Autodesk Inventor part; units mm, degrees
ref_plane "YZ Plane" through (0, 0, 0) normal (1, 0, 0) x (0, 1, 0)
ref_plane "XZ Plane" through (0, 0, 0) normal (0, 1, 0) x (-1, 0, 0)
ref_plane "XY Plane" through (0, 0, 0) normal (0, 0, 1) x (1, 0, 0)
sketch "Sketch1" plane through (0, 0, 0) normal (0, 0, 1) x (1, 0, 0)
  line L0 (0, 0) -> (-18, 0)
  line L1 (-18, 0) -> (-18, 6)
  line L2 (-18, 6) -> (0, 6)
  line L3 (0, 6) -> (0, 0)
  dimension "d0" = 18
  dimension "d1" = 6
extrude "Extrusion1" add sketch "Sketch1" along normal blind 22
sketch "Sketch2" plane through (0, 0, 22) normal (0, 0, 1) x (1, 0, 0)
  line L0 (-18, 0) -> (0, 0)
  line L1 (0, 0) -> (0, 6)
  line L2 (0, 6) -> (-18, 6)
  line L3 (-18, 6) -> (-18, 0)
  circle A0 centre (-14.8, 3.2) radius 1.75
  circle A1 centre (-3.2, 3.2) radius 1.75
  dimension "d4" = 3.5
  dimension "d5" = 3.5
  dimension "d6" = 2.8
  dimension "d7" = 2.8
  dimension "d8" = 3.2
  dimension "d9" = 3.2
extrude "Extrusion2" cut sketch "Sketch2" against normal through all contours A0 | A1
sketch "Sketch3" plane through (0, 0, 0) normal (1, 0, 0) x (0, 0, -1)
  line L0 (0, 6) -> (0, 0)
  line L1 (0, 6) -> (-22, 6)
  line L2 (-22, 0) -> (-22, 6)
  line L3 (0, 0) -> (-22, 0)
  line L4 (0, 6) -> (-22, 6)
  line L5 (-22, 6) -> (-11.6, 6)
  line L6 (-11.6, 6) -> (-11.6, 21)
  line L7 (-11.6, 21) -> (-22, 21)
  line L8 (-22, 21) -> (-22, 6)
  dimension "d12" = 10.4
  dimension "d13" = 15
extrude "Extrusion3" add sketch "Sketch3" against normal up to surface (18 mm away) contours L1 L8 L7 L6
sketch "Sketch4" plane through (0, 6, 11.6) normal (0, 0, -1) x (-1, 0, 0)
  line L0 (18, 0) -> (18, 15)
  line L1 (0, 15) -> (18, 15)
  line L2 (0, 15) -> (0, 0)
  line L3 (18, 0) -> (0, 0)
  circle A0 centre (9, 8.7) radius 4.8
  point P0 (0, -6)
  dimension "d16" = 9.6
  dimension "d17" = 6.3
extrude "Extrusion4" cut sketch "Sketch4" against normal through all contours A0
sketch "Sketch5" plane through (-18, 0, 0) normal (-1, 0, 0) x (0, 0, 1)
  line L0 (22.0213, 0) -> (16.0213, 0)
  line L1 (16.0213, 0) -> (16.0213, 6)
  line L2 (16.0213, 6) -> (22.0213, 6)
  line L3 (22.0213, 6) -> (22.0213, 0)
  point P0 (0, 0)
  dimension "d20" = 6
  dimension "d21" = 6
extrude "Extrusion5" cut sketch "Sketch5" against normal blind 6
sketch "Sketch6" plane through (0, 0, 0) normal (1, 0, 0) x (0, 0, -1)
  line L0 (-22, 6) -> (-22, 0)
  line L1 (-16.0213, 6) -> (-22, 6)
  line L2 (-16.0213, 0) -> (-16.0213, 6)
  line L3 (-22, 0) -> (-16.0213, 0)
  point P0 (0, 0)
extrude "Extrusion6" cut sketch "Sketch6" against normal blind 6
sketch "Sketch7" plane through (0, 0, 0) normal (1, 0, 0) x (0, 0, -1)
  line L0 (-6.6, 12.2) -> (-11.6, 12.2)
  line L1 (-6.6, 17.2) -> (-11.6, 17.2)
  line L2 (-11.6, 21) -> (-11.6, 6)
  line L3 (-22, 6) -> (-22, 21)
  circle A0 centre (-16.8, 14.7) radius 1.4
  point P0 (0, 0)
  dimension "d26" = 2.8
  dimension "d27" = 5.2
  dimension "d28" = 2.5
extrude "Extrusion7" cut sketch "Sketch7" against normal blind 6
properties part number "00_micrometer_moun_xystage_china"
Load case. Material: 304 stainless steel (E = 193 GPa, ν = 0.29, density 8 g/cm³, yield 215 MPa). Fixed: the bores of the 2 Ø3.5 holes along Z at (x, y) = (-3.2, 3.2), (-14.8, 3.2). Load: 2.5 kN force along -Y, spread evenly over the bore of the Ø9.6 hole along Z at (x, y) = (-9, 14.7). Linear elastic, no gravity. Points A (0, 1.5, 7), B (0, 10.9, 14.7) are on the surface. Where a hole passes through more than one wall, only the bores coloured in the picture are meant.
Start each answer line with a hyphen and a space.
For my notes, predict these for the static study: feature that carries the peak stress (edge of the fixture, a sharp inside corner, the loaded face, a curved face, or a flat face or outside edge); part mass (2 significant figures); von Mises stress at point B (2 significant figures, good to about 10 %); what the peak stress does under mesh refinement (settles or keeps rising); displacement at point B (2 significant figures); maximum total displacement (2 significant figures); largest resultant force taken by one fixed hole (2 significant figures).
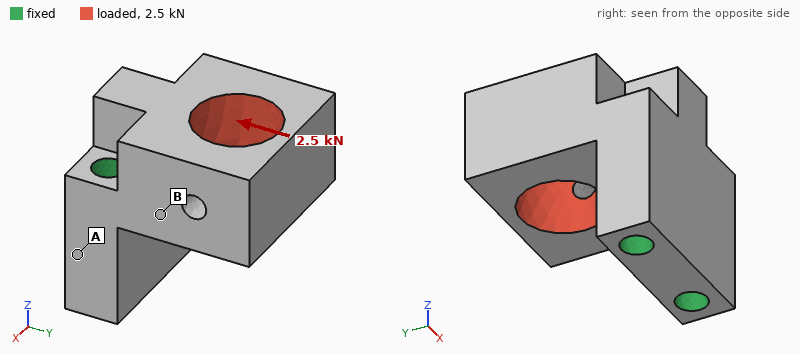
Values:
- edge of the fixture
- 29 g
- 25 MPa
- keeps rising
- 3.7 µm
- 15 µm
- 1.3 kN
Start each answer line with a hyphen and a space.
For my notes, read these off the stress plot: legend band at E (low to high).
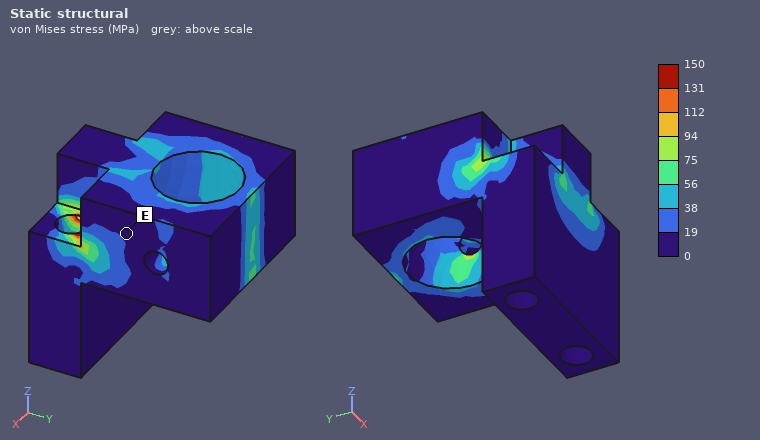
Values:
- 0 to 19 MPa
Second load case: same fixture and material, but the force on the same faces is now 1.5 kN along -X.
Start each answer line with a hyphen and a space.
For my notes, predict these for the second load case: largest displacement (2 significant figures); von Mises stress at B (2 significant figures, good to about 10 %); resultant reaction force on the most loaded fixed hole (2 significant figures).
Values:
- 11 µm
- 46 MPa
- 1.5 kN
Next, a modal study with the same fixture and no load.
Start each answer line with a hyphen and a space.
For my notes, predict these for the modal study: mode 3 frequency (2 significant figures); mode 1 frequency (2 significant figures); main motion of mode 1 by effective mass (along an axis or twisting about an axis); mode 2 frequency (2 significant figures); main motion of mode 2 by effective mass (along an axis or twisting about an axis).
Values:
- 25 kHz
- 12 kHz
- along Z
- 19 kHz
- along X
